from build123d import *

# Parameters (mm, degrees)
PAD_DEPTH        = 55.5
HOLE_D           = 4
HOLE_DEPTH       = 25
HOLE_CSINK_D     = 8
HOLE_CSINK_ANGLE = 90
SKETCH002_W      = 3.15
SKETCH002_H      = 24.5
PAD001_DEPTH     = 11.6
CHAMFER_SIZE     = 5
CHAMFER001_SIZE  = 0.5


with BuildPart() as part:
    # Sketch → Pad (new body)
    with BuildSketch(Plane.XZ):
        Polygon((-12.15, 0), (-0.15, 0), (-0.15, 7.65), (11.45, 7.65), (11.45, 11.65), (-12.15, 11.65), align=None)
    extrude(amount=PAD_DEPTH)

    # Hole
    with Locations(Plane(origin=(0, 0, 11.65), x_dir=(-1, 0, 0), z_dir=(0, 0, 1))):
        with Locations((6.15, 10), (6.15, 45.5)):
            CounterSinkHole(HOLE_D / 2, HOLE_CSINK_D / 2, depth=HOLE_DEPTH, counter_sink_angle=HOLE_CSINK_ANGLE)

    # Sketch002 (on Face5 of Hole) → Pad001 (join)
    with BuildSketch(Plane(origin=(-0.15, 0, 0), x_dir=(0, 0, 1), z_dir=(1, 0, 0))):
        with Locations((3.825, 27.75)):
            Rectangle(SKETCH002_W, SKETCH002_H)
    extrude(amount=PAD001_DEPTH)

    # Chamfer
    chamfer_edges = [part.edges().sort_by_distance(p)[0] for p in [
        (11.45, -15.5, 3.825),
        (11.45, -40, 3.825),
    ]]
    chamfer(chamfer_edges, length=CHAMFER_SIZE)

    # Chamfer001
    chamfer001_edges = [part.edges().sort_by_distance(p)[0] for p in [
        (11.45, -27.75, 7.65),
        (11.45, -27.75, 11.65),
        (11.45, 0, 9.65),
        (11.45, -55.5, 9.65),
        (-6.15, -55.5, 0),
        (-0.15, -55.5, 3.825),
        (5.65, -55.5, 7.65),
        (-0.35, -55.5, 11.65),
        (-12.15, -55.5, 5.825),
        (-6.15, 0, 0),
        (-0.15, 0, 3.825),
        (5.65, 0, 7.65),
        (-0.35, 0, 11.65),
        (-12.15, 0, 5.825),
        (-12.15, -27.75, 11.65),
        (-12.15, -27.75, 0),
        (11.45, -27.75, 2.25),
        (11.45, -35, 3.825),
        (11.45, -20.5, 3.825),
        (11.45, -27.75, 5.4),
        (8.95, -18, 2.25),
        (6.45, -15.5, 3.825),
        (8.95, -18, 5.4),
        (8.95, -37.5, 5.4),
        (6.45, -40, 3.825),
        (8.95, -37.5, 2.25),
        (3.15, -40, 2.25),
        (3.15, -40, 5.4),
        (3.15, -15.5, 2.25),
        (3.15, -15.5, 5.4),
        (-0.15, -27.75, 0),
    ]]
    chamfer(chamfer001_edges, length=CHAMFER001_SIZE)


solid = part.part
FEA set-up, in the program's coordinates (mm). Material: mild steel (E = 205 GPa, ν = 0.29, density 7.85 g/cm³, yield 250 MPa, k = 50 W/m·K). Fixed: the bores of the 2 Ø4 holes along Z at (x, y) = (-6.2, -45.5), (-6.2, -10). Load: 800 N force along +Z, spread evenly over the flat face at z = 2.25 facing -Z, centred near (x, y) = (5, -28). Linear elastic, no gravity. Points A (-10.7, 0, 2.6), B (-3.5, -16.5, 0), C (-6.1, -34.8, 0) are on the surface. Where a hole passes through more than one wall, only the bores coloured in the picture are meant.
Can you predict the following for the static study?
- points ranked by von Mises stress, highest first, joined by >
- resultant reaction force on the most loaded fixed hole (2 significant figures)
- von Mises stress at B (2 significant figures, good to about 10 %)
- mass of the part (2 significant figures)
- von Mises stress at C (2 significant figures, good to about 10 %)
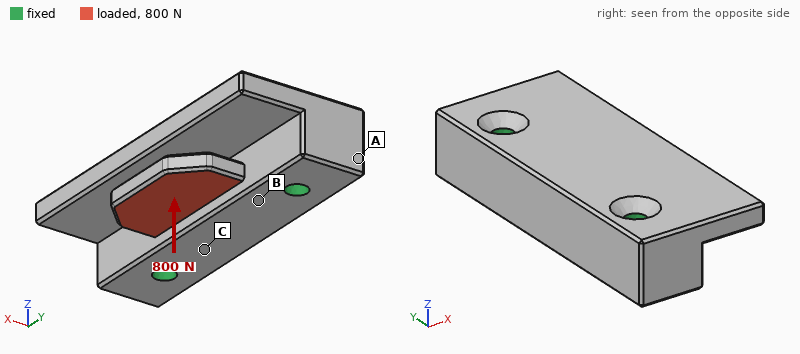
B > C > A
400 N
24 MPa
84 g
15 MPa
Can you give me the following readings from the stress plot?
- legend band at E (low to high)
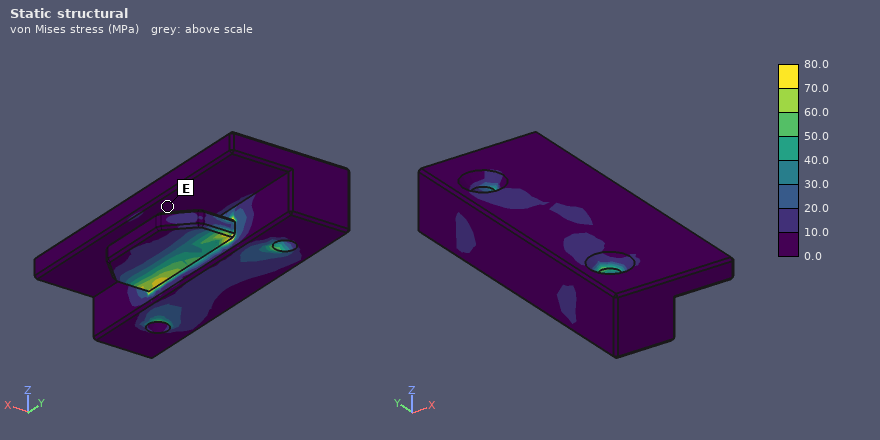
0.0 to 10.0 MPa
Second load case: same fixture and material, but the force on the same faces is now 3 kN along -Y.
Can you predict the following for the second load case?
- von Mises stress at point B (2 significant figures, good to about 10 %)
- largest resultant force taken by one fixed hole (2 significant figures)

20 MPa
1.8 kN
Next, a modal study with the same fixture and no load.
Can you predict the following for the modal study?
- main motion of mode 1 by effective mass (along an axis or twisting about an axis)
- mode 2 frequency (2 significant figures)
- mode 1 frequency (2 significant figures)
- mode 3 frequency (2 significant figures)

along Z
17 kHz
13 kHz
18 kHz
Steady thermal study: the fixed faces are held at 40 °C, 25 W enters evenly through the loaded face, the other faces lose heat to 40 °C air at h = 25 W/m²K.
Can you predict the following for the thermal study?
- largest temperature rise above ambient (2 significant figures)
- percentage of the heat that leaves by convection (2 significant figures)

64 K
4.9 %
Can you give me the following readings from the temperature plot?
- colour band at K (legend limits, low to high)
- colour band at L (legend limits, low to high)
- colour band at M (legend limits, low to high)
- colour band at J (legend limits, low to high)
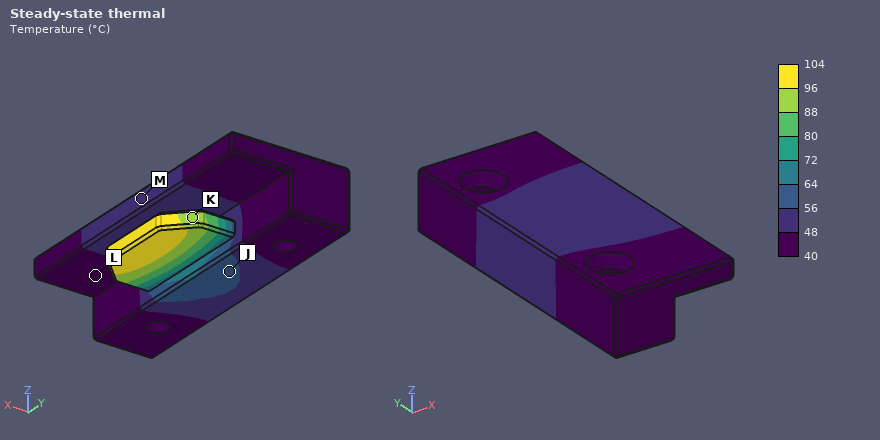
88 to 96 °C
40 to 48 °C
48 to 56 °C
56 to 64 °C
